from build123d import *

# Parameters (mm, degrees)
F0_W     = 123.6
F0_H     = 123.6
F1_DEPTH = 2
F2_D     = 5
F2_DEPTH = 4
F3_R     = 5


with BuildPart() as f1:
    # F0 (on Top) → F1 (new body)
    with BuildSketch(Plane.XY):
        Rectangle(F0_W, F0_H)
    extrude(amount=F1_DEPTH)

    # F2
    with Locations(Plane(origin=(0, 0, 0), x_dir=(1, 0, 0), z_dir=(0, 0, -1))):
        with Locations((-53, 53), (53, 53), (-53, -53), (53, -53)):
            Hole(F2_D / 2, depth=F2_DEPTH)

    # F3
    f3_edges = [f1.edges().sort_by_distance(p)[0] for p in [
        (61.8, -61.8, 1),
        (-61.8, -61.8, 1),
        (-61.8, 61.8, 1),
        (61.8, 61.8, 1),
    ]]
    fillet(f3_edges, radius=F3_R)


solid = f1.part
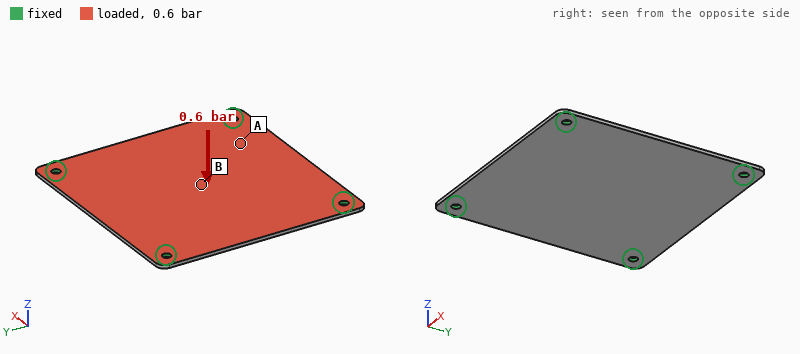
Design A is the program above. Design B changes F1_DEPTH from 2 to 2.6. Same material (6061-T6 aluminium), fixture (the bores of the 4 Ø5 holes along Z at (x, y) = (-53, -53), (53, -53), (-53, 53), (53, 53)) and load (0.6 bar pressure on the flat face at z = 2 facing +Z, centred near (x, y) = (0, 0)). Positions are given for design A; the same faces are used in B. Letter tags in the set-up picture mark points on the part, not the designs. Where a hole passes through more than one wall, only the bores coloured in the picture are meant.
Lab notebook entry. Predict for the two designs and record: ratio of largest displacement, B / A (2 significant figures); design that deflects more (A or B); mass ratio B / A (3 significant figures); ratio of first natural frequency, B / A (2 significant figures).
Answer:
0.46
A
1.30
1.3
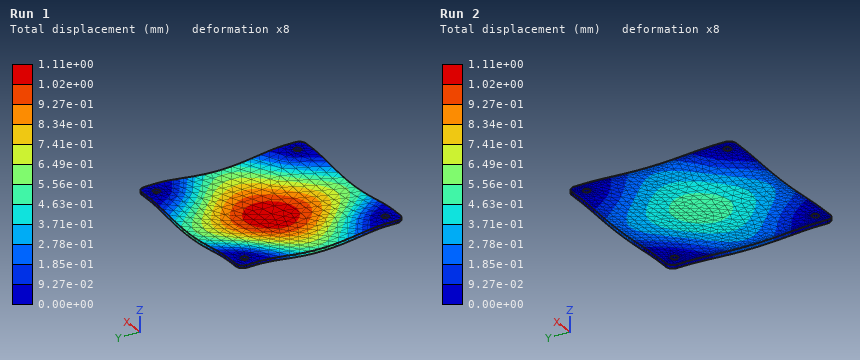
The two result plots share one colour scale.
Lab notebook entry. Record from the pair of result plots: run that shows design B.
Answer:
Run 2
